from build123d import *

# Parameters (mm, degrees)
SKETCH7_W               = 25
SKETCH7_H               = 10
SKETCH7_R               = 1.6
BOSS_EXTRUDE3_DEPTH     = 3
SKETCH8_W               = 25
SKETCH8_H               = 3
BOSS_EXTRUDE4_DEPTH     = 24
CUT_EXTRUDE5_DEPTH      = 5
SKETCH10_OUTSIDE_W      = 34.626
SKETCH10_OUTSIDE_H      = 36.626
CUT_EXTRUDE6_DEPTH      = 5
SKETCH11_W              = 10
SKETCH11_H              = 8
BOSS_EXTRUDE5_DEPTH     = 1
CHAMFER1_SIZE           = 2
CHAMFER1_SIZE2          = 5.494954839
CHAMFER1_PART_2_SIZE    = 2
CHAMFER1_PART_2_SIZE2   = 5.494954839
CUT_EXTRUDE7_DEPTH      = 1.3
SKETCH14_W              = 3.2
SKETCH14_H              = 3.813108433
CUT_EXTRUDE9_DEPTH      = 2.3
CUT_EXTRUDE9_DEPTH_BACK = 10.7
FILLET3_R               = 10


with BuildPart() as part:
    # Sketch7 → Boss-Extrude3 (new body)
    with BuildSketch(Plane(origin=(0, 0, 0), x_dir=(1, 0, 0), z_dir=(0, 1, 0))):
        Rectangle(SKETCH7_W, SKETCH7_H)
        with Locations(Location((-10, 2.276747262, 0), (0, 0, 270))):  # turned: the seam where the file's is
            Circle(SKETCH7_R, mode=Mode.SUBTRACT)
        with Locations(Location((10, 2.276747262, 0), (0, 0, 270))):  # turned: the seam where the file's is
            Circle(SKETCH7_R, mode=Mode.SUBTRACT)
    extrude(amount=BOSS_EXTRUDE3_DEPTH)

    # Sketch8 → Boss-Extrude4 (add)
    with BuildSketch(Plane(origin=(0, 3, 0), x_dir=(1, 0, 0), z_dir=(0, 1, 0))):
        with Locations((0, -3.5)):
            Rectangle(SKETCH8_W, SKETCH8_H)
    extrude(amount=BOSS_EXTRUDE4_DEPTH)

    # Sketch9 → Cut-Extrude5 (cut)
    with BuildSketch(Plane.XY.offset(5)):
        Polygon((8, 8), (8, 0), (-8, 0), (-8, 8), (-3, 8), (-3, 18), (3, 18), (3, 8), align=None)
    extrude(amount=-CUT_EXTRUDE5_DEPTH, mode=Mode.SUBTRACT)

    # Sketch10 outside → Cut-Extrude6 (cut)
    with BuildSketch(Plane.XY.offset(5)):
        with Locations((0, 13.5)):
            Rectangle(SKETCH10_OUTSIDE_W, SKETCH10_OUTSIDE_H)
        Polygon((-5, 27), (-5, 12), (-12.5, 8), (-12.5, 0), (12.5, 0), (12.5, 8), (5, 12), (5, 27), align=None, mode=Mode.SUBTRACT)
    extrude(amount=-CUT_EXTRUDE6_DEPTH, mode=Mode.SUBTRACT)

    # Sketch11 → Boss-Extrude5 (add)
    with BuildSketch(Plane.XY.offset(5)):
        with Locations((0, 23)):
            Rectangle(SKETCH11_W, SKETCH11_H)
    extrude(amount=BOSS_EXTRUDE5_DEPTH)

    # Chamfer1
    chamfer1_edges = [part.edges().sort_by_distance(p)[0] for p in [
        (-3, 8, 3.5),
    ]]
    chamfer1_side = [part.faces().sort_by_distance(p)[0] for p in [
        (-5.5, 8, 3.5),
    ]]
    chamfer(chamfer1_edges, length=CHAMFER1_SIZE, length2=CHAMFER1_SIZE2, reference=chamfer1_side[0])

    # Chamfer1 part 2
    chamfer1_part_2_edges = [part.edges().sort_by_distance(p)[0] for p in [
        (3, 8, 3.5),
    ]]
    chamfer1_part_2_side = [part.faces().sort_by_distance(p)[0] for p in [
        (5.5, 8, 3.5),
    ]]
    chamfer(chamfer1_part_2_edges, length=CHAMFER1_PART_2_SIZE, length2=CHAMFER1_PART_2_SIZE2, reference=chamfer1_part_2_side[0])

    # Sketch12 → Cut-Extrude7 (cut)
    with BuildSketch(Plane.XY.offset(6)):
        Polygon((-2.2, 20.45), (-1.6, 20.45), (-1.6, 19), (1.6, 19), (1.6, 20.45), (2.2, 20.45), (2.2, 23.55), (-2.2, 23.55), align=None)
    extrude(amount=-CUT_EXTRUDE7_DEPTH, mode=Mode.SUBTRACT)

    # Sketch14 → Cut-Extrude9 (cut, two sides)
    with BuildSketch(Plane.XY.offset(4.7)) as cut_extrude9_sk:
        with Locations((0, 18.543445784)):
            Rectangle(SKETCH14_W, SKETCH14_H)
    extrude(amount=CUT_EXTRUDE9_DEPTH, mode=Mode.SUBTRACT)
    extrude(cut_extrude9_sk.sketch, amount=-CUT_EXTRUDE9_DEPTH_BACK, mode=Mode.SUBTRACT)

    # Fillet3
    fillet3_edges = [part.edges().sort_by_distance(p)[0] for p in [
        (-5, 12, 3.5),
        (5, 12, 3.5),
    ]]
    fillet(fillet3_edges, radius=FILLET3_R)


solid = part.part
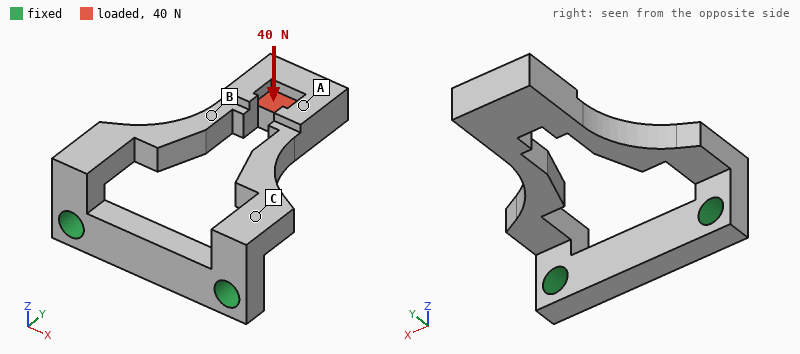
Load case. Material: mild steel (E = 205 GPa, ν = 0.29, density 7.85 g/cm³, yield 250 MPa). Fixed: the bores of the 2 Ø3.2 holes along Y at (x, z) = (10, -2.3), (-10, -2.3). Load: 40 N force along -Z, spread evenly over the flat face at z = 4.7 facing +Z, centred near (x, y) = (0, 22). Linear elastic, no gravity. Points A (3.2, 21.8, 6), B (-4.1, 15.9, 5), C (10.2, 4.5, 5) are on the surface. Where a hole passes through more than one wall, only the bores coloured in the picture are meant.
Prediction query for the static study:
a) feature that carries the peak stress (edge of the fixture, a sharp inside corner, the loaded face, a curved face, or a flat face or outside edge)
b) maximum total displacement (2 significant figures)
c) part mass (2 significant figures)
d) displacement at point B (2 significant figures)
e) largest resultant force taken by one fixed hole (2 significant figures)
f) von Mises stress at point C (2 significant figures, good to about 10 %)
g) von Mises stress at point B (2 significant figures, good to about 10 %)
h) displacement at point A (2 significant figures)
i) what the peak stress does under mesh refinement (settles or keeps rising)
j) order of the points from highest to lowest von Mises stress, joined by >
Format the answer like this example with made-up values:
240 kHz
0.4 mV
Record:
a sharp inside corner
81 µm
8.7 g
36 µm
20 N
55 MPa
38 MPa
60 µm
keeps rising
C > B > A
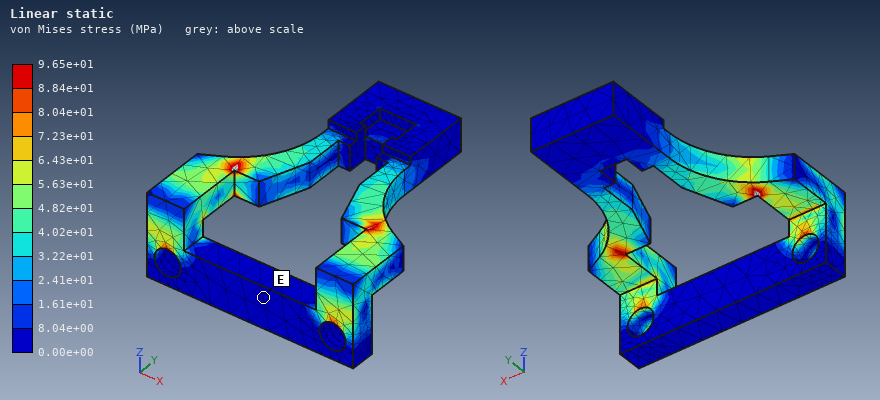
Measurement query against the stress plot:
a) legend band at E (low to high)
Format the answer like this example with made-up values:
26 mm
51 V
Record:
0.00e+00 to 8.04e+00 MPa
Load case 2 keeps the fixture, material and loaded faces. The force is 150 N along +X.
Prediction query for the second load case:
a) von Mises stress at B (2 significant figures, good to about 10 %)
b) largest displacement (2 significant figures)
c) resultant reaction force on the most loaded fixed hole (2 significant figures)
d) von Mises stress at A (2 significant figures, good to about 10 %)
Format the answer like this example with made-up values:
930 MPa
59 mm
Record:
56 MPa
15 µm
140 N
16 MPa
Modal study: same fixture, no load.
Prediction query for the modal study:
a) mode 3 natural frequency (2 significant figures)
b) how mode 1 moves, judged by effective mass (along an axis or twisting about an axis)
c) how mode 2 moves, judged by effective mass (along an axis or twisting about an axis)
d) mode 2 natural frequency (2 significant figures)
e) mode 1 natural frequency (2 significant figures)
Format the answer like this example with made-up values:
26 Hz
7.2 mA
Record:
11 kHz
along Z
along X
9200 Hz
2400 Hz
